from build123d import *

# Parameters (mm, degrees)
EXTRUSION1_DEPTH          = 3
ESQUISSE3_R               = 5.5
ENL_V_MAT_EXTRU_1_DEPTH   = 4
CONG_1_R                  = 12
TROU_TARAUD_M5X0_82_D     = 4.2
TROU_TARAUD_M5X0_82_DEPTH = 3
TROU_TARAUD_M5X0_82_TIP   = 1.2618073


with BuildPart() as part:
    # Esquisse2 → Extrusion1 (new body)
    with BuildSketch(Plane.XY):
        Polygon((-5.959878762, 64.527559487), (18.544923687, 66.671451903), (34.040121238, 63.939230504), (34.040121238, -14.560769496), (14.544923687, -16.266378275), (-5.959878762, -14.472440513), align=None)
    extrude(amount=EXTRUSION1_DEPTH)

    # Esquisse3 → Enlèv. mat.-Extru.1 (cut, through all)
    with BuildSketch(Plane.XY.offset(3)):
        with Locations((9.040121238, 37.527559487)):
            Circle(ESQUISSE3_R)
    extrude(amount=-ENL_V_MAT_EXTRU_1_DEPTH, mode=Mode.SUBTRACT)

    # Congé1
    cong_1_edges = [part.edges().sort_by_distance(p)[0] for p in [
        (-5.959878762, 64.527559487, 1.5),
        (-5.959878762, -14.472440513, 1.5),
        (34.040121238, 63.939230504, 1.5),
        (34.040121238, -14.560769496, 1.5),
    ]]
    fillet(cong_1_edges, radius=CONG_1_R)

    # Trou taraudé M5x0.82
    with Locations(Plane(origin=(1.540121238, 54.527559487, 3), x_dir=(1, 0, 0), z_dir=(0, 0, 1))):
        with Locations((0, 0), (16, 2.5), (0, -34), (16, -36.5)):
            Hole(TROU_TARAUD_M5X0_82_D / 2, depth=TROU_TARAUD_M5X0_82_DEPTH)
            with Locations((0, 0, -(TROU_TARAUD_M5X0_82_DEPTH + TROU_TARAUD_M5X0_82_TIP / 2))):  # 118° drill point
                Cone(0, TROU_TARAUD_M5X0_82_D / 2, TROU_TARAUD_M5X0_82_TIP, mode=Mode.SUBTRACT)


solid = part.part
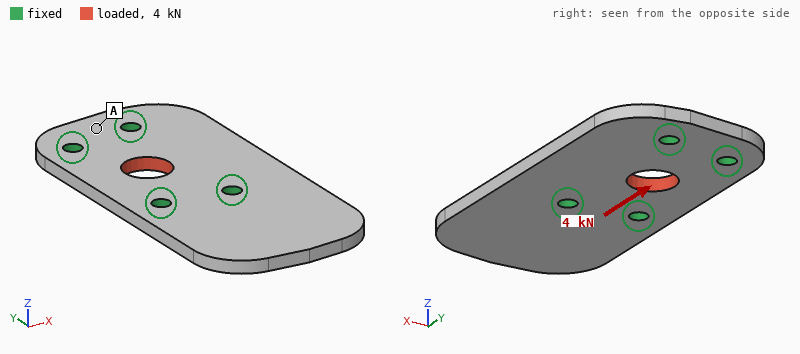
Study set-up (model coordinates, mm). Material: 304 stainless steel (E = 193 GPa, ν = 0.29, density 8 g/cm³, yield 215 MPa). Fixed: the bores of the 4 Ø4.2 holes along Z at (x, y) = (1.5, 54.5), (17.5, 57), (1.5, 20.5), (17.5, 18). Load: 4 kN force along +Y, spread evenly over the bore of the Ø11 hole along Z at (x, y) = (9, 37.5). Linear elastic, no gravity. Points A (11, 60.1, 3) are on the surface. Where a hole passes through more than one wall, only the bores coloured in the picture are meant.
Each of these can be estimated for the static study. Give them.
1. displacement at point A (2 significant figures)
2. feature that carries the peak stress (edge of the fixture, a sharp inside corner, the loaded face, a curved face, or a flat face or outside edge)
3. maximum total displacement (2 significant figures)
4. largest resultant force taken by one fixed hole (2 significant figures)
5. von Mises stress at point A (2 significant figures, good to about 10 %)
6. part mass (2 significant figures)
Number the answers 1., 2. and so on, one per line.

1. 0.43 µm
2. the loaded face
3. 2.8 µm
4. 1.1 kN
5. 7.9 MPa
6. 72 g
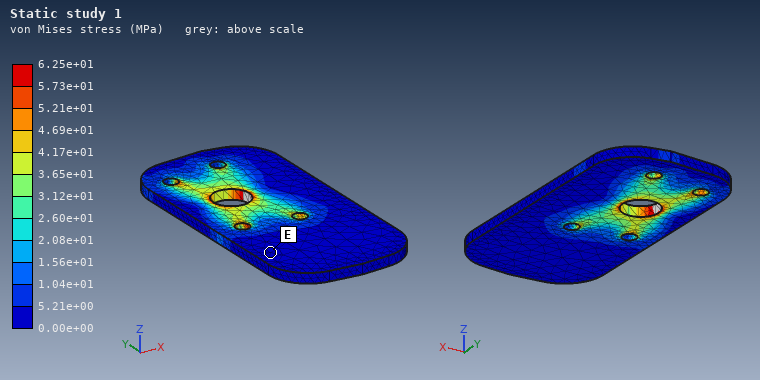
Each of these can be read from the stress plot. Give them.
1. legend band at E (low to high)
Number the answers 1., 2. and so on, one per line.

1. 0.00e+00 to 5.21e+00 MPa
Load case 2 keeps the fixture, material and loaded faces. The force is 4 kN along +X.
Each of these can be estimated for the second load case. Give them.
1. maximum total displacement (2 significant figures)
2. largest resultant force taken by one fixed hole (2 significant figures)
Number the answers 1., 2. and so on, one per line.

1. 6.2 µm
2. 1.2 kN
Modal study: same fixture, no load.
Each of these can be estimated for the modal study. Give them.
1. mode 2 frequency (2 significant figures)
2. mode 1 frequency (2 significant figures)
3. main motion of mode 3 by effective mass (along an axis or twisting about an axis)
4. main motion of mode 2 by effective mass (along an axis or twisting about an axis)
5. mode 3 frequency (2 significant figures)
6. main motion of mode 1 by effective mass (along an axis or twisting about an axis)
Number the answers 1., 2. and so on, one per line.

1. 4500 Hz
2. 2200 Hz
3. along Z
4. twisting about Y
5. 7000 Hz
6. along Z
